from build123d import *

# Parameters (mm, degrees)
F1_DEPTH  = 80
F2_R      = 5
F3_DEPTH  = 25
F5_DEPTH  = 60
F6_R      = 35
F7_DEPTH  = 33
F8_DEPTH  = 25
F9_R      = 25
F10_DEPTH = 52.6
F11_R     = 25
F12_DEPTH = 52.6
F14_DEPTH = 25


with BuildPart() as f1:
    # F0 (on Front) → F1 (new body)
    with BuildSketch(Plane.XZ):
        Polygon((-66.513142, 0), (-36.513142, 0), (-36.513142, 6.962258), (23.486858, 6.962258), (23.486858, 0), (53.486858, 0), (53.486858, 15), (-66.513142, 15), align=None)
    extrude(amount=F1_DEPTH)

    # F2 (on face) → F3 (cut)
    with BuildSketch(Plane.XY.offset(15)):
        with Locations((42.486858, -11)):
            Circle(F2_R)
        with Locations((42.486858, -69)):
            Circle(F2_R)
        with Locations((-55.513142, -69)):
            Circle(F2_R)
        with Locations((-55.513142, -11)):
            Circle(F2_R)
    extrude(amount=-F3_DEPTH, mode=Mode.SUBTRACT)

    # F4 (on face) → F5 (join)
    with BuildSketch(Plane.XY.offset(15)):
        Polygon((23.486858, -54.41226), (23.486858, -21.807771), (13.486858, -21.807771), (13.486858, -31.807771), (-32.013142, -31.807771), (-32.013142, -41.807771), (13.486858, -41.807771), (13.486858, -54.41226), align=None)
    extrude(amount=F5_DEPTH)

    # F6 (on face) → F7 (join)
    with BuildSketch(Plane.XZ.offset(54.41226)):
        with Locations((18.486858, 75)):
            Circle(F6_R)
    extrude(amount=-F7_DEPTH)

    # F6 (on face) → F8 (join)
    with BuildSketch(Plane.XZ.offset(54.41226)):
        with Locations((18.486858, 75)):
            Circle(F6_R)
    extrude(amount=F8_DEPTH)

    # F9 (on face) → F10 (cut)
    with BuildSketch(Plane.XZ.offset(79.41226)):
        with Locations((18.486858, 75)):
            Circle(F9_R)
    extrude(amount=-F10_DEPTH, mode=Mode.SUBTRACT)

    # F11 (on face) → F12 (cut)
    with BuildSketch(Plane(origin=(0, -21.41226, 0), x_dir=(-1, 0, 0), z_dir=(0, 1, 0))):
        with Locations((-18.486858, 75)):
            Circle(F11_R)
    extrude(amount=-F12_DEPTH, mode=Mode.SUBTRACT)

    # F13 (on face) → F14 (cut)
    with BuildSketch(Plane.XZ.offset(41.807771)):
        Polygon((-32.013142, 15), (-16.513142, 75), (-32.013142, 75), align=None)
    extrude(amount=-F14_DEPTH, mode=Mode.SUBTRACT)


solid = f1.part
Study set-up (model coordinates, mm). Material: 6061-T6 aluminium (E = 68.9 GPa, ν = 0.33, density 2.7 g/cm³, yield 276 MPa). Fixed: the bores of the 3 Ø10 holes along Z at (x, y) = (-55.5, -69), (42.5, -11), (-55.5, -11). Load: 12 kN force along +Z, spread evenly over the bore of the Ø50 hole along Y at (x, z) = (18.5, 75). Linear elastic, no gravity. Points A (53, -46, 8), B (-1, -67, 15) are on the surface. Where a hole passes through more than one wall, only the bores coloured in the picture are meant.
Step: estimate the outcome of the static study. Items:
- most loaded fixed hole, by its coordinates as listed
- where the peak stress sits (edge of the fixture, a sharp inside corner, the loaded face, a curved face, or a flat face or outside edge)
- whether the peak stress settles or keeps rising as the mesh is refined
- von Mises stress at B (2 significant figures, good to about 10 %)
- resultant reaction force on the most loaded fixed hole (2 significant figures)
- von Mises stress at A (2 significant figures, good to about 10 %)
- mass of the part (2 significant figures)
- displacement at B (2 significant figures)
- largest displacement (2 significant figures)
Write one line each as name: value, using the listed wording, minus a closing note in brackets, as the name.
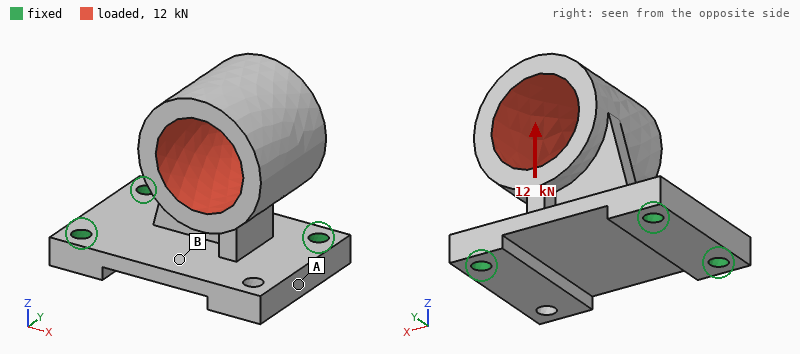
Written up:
most loaded fixed hole, by its coordinates as listed: (42.5, -11)
where the peak stress sits: edge of the fixture
whether the peak stress settles or keeps rising as the mesh is refined: keeps rising
von Mises stress at B: 67 MPa
resultant reaction force on the most loaded fixed hole: 10 kN
von Mises stress at A: 22 MPa
mass of the part: 640 g
displacement at B: 0.26 mm
largest displacement: 1.1 mm
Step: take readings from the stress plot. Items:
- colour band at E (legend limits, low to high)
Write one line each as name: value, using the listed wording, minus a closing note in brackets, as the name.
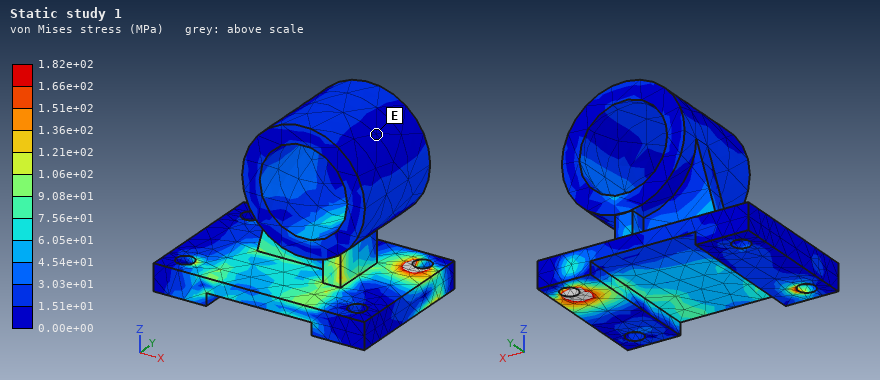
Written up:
colour band at E: 0.00e+00 to 1.51e+01 MPa
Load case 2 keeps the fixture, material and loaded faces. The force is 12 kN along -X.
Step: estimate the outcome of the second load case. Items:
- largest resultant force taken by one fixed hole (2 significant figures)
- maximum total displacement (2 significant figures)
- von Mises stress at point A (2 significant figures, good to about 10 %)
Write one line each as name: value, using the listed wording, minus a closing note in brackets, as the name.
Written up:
largest resultant force taken by one fixed hole: 12 kN
maximum total displacement: 0.93 mm
von Mises stress at point A: 26 MPa
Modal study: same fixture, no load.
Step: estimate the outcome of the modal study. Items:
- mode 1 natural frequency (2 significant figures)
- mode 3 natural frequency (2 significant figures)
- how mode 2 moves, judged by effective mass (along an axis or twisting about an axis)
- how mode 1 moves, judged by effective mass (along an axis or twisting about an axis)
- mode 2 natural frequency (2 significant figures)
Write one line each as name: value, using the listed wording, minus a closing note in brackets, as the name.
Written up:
mode 1 natural frequency: 660 Hz
mode 3 natural frequency: 1900 Hz
how mode 2 moves, judged by effective mass: along X
how mode 1 moves, judged by effective mass: along Y
mode 2 natural frequency: 1200 Hz
